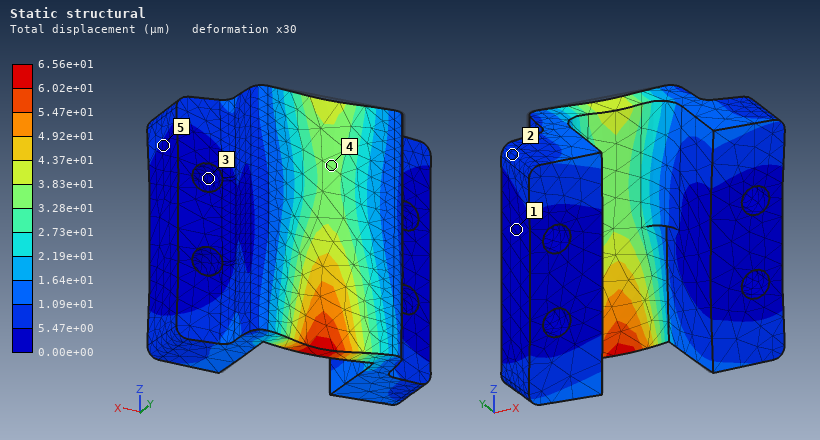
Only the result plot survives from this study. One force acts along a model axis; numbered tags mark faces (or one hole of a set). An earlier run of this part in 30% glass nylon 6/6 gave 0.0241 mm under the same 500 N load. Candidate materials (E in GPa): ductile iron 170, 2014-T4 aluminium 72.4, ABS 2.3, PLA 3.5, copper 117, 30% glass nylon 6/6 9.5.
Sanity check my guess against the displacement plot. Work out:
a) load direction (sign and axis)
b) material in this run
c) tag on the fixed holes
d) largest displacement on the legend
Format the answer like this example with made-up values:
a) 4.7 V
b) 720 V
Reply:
a) -Y
b) PLA
c) 3
d) 6.56e+01 µm
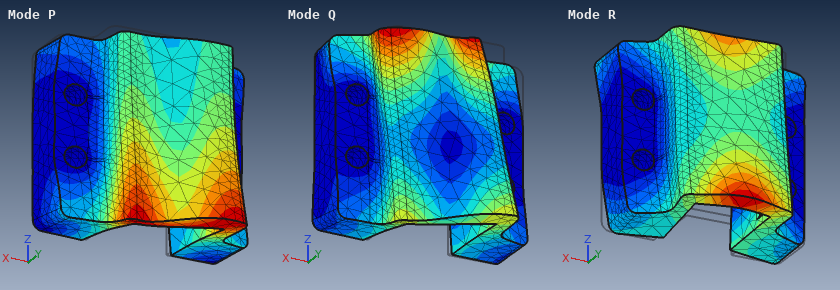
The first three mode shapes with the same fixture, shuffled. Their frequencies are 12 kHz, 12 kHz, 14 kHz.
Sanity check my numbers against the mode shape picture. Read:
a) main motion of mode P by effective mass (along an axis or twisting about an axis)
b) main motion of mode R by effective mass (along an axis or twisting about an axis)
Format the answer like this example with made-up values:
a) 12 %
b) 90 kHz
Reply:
a) along X
b) along Z
